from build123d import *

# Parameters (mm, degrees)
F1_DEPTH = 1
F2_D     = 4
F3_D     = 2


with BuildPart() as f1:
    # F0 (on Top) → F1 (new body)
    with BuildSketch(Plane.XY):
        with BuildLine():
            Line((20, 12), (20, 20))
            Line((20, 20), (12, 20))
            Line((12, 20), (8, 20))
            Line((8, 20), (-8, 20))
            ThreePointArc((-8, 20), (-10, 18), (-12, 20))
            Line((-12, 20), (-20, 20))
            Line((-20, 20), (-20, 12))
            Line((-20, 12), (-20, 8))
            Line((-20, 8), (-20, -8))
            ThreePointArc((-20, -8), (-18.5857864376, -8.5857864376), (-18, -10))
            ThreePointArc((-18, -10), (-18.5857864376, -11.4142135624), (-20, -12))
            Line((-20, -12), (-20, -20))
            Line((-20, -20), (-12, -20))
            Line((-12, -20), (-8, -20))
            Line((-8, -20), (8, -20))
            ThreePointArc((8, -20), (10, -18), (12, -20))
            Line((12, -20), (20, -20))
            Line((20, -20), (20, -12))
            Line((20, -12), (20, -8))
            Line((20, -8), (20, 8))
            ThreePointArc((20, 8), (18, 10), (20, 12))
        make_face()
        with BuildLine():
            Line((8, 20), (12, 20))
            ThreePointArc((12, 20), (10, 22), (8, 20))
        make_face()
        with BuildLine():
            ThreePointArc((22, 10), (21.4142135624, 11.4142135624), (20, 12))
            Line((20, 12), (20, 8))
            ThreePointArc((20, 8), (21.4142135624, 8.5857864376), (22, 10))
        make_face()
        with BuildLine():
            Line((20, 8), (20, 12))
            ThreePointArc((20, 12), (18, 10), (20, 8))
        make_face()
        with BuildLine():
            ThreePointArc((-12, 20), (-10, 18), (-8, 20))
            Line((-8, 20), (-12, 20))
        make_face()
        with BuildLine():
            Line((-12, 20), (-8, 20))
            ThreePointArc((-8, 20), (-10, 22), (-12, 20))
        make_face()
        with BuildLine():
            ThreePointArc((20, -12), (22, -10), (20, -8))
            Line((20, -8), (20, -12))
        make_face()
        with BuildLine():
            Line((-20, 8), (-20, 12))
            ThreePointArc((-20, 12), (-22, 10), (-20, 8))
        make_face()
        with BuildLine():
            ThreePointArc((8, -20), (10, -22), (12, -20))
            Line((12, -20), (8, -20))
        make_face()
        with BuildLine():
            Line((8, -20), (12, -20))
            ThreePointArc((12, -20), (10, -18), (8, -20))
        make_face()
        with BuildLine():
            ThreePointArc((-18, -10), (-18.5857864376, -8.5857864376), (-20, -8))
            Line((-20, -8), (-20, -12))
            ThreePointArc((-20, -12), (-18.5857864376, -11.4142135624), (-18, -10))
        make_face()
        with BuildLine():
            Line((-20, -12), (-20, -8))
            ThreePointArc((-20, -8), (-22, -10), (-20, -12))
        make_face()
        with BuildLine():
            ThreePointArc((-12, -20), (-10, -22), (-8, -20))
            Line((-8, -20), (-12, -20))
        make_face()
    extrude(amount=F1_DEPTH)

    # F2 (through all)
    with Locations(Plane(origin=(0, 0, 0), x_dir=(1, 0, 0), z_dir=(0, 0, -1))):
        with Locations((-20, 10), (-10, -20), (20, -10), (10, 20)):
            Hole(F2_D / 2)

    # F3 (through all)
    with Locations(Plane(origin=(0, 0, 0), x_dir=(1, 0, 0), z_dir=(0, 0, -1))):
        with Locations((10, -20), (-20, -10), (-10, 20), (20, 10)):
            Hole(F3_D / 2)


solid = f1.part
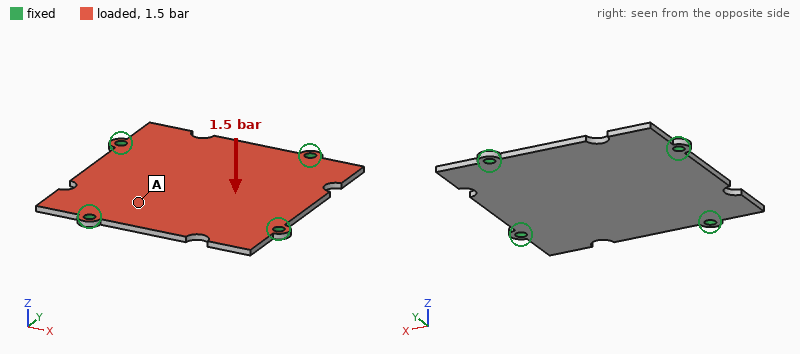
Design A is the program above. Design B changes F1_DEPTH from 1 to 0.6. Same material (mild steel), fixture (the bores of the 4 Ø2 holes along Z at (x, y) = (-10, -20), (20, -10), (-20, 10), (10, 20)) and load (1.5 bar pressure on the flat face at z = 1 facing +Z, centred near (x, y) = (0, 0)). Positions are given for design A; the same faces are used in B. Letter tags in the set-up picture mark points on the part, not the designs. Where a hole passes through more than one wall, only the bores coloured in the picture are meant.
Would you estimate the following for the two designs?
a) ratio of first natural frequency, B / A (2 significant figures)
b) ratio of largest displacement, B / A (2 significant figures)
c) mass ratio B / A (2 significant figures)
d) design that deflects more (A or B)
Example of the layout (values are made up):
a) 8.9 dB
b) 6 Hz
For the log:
a) 0.61
b) 4.4
c) 0.60
d) B
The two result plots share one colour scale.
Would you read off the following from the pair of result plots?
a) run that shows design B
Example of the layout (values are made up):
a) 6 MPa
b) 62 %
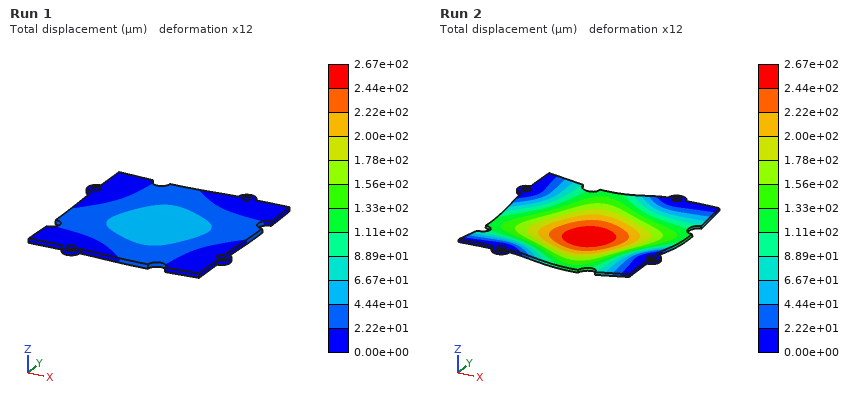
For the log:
a) Run 2
